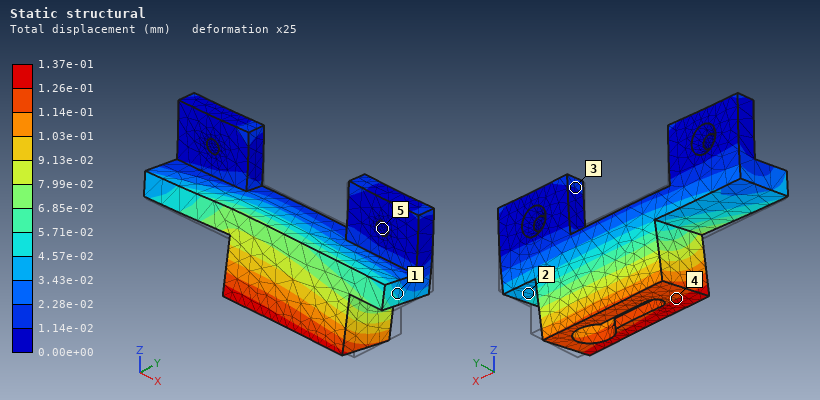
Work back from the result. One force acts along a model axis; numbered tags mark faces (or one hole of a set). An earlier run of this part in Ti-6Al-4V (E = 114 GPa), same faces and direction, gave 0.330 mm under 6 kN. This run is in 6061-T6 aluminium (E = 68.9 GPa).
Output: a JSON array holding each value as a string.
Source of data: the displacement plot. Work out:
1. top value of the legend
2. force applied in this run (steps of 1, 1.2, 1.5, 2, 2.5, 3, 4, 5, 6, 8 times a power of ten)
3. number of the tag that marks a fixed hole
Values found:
["1.37e-01 mm", "1.5 kN", "5"]
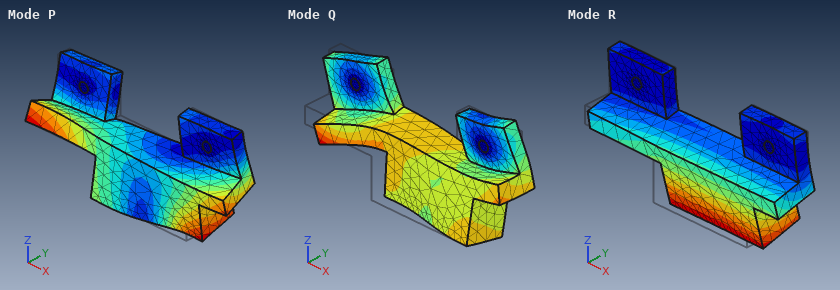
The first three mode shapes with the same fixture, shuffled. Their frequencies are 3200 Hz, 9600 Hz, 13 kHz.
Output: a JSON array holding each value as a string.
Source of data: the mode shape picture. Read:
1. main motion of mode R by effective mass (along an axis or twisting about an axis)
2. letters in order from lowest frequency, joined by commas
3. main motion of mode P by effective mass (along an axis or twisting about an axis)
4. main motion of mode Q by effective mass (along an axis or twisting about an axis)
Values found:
["along Y", "R, P, Q", "twisting about Z", "along X"]
